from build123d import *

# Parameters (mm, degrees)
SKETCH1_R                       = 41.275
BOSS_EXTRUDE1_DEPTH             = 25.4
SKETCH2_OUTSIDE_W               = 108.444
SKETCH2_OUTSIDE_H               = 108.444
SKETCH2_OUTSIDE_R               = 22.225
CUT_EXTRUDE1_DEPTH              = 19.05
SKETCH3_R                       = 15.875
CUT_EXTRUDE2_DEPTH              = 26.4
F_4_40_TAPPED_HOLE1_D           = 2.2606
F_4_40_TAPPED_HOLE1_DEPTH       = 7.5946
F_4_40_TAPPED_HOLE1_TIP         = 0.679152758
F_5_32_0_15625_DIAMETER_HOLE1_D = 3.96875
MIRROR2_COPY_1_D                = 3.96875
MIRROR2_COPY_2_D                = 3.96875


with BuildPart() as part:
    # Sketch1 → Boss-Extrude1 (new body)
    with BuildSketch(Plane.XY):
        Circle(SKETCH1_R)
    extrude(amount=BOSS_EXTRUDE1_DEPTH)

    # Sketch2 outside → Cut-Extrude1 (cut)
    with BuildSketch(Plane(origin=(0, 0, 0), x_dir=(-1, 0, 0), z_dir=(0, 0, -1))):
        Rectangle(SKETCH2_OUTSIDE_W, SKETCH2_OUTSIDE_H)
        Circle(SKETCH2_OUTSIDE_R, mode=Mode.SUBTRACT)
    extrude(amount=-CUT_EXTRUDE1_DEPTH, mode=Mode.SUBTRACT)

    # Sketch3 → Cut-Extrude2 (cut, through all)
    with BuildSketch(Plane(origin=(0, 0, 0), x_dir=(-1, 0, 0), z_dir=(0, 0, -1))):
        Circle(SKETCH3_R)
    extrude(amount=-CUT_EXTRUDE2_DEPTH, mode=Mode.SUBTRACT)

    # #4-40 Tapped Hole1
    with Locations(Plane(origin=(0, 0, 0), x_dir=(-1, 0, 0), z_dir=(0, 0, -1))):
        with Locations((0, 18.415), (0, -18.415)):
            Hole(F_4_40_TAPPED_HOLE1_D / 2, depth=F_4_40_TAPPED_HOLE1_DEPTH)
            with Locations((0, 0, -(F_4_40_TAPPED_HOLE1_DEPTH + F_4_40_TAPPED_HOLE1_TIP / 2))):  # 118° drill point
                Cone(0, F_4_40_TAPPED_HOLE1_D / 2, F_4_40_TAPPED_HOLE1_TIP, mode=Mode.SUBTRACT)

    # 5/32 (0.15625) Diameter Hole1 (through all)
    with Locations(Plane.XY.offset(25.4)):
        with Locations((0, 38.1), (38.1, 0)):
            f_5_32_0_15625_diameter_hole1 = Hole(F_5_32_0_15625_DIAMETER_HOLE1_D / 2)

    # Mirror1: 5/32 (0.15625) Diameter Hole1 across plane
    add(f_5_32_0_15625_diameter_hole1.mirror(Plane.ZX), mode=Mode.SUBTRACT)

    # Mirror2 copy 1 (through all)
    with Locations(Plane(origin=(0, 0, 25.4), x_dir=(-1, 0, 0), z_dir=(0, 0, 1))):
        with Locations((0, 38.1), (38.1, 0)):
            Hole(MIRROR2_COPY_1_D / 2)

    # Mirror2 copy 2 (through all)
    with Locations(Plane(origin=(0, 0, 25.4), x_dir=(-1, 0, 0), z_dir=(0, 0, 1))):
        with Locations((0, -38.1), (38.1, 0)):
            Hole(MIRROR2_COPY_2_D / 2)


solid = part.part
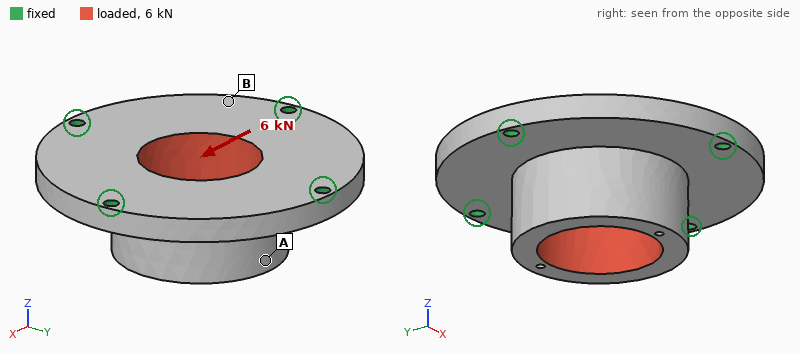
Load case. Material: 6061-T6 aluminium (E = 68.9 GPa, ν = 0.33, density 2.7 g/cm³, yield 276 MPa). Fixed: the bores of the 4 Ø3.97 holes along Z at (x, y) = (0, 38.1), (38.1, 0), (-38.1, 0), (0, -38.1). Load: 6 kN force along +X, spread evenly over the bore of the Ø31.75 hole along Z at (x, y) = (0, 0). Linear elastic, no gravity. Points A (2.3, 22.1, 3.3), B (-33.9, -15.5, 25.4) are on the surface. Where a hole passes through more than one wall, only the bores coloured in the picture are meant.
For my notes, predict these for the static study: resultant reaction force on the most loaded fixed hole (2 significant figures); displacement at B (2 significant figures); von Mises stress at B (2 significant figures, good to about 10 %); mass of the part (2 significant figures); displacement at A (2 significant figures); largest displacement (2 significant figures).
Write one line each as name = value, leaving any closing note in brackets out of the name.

resultant reaction force on the most loaded fixed hole = 2.0 kN
displacement at B = 9.0 µm
von Mises stress at B = 11 MPa
mass of the part = 120 g
displacement at A = 20 µm
largest displacement = 28 µm
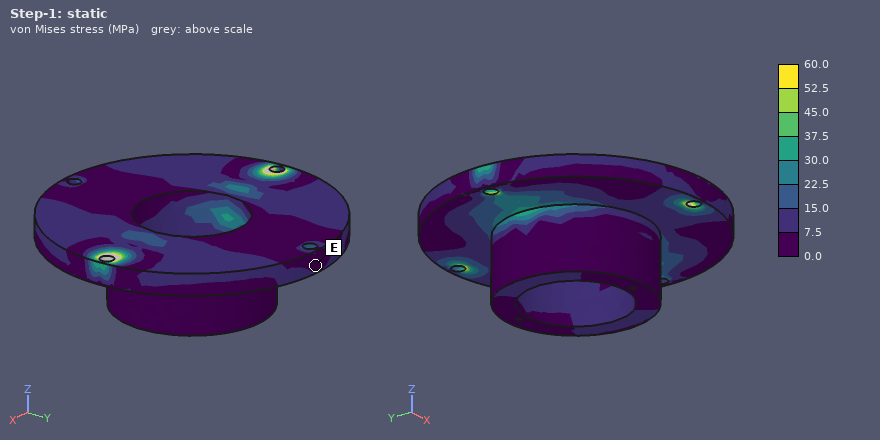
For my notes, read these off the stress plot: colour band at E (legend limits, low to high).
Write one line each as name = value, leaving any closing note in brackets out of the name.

colour band at E = 0.0 to 7.5 MPa
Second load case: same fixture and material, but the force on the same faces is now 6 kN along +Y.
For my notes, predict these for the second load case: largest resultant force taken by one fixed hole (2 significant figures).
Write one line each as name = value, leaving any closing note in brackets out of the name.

largest resultant force taken by one fixed hole = 2.0 kN
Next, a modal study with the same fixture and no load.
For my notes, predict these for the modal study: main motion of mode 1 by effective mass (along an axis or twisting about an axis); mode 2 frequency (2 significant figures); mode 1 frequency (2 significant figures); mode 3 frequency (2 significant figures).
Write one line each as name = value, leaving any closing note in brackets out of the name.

main motion of mode 1 by effective mass = along Z
mode 2 frequency = 8300 Hz
mode 1 frequency = 7200 Hz
mode 3 frequency = 8300 Hz
